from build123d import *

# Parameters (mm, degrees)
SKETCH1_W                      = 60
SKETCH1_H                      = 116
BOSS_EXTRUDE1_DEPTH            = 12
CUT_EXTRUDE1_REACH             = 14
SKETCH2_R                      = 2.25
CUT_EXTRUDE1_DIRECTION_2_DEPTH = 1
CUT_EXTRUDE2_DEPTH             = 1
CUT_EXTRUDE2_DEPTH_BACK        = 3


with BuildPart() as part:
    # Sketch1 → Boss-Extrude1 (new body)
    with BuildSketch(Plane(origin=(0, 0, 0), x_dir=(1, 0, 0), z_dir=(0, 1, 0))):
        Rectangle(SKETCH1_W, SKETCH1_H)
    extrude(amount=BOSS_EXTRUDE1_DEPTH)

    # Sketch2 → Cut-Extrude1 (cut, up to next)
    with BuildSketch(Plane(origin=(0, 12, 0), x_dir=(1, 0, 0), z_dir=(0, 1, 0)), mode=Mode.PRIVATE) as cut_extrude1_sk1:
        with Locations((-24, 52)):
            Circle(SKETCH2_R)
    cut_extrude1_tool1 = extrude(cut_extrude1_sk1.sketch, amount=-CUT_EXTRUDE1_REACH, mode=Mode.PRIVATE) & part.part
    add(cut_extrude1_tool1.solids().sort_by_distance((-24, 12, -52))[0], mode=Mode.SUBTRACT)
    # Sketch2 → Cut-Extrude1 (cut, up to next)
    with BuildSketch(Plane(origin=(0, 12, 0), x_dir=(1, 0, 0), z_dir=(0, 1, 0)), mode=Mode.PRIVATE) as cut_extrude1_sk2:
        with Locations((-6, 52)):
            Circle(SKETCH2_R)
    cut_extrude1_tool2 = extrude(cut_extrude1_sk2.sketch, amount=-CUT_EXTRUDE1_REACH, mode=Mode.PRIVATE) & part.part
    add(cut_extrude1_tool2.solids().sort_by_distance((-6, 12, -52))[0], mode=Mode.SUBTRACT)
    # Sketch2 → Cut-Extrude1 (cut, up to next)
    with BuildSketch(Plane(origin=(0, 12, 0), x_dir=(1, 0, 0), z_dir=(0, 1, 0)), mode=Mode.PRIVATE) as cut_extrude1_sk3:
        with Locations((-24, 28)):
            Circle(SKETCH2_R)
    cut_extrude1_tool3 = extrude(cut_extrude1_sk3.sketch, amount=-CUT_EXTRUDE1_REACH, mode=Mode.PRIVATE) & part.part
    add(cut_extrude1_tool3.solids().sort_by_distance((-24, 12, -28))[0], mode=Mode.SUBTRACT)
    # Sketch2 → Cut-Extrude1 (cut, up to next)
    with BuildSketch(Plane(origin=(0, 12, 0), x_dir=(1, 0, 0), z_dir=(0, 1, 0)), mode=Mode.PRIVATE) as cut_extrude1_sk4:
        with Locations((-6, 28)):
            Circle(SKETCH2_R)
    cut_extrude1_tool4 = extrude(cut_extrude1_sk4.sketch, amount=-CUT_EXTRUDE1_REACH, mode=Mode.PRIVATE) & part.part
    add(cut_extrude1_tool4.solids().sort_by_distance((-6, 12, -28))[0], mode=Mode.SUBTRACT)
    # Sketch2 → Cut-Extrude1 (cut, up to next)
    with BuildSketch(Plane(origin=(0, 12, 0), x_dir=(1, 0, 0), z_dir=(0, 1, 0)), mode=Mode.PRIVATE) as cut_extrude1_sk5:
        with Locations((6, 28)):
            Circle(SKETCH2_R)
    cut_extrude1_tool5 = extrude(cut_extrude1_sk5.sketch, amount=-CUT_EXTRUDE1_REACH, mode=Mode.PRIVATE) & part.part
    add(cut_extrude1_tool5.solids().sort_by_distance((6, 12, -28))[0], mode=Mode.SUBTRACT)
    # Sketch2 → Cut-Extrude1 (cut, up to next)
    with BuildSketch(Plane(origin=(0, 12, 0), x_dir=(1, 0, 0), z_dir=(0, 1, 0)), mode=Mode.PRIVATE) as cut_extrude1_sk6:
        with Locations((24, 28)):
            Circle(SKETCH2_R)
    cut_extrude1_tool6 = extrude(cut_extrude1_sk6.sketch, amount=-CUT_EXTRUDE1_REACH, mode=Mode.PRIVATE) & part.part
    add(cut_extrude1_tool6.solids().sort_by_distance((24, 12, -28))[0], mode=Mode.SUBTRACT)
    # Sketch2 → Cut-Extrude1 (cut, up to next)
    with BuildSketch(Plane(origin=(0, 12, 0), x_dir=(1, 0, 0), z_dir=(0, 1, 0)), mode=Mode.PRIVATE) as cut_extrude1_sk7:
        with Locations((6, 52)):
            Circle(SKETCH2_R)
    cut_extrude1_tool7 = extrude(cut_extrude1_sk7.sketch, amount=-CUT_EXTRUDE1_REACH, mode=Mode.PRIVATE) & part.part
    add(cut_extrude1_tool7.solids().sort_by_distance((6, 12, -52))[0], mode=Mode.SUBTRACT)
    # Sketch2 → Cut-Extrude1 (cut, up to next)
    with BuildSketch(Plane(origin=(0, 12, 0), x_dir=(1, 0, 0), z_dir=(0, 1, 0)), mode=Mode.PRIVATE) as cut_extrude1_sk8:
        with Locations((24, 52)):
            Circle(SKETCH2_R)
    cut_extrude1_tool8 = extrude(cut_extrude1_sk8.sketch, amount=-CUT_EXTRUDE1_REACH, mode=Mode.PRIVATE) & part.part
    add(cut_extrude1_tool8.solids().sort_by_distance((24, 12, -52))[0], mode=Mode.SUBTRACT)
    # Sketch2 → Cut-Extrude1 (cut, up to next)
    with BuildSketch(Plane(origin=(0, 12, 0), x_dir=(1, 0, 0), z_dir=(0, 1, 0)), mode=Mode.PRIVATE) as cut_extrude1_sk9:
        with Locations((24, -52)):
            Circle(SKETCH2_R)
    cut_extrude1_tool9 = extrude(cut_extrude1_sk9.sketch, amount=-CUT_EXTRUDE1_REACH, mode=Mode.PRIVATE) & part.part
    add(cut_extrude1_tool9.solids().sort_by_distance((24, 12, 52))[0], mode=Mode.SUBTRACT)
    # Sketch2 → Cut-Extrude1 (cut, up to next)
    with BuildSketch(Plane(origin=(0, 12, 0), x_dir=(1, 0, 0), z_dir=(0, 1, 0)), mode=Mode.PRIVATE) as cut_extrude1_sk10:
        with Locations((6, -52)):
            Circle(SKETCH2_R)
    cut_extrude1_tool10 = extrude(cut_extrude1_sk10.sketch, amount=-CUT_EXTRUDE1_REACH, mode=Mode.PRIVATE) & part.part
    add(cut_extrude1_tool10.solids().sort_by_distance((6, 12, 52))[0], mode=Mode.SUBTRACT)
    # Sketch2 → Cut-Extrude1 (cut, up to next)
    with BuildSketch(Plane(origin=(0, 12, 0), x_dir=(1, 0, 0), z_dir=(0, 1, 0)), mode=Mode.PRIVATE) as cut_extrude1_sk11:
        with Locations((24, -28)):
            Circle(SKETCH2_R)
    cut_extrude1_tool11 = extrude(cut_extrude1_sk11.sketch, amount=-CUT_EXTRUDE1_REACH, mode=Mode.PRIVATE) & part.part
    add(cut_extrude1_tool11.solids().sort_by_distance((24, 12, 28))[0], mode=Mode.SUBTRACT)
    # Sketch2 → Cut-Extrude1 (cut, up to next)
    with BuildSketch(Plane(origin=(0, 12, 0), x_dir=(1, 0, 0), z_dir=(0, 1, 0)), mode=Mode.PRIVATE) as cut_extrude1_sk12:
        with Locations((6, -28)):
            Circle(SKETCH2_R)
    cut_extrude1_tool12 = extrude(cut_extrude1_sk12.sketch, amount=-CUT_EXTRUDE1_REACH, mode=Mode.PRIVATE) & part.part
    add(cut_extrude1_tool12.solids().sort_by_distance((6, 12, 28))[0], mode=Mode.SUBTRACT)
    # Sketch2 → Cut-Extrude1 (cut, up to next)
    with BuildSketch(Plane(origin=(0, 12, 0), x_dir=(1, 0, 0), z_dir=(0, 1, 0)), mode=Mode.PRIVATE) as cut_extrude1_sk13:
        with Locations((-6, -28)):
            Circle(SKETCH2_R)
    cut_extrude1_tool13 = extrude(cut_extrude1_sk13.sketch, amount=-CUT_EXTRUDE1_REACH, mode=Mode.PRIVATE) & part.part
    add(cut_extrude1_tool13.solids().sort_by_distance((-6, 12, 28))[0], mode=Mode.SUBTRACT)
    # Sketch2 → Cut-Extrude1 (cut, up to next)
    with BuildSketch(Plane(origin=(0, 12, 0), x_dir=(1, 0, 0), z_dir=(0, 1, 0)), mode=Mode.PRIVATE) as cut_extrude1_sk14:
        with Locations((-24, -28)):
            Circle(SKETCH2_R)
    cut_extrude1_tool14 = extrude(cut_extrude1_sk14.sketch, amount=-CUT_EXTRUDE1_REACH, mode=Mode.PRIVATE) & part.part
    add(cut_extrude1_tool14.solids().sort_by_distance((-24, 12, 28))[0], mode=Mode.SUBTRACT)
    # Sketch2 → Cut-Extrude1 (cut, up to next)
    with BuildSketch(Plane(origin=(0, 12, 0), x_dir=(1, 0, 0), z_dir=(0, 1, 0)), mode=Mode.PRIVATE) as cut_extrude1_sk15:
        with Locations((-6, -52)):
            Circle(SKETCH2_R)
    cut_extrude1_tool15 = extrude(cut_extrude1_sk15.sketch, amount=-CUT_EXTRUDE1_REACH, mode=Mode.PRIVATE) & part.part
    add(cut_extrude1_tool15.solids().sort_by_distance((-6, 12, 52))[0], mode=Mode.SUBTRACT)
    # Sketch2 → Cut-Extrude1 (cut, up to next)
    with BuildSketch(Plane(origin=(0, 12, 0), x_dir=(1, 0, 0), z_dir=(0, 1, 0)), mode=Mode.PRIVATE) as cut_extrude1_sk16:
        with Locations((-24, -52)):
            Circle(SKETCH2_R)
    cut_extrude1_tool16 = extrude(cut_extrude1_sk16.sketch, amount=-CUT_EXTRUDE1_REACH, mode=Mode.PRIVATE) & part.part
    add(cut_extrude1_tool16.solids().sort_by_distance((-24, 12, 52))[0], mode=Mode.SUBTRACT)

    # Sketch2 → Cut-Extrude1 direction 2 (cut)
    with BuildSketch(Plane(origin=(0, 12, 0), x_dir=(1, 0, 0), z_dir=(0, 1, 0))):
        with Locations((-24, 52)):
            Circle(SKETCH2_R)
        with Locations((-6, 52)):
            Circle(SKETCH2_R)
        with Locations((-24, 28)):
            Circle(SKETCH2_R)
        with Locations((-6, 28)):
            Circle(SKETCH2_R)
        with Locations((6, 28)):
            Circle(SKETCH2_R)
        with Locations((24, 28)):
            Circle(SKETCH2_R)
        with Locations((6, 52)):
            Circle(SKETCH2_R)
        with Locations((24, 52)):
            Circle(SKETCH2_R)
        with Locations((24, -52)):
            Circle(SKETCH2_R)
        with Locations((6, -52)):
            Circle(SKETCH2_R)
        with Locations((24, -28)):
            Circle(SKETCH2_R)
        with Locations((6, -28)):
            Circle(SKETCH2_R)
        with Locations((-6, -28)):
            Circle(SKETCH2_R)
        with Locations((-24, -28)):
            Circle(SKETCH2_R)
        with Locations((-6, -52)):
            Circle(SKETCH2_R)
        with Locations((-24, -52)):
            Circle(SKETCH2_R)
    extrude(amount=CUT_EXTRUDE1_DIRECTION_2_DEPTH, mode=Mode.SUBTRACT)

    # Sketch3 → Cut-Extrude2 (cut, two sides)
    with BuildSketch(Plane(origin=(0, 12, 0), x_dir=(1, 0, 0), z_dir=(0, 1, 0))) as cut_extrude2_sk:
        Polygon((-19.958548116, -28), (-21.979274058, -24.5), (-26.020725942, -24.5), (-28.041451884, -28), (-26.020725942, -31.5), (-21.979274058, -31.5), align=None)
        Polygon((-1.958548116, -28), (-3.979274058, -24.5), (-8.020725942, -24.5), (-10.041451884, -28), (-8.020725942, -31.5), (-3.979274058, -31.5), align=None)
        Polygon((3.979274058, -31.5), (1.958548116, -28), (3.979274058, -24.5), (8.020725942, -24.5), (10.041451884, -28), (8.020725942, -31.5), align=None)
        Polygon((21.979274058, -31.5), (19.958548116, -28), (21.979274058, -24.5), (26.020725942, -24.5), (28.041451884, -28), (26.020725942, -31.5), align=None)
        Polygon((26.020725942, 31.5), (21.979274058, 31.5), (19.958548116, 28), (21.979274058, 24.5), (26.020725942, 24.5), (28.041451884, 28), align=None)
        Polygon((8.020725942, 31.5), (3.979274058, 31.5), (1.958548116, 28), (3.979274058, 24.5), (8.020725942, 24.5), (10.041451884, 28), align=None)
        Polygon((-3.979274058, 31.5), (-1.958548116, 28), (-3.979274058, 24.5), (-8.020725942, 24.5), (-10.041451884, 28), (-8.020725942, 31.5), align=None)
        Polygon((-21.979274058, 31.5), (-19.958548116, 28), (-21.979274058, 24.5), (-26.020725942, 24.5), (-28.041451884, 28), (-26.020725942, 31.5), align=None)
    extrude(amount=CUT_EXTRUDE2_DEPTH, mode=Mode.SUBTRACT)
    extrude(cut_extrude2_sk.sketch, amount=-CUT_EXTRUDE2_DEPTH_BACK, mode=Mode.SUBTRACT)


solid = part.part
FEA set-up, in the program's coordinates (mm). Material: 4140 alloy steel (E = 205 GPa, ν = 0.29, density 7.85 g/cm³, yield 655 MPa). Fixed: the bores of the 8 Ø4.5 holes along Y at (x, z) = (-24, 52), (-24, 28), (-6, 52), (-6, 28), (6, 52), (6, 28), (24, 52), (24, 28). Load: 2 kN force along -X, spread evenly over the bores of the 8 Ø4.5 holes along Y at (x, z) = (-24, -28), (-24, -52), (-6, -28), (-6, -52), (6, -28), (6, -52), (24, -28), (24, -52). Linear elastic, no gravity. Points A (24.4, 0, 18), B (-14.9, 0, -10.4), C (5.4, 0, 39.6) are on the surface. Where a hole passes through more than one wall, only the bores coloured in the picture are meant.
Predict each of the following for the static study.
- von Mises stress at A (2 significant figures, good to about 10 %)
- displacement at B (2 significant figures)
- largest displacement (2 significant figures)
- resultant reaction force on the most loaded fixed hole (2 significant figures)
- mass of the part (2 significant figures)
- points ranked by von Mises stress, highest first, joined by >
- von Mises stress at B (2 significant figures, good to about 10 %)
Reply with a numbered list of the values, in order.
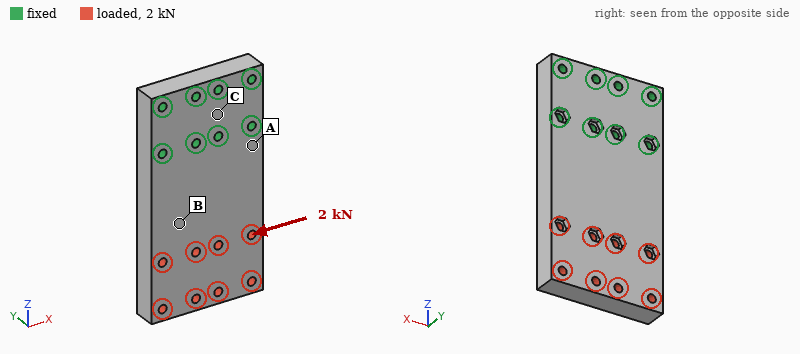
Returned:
1. 17 MPa
2. 4.1 µm
3. 12 µm
4. 2.4 kN
5. 630 g
6. A > B > C
7. 7.7 MPa
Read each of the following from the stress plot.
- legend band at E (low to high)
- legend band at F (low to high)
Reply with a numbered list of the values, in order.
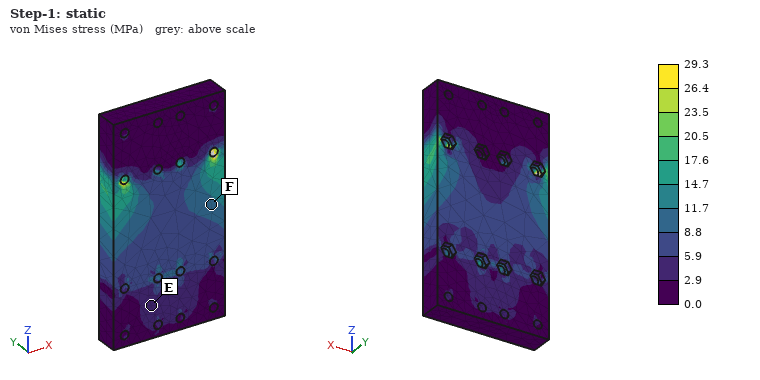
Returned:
1. 2.9 to 5.9 MPa
2. 8.8 to 11.7 MPa
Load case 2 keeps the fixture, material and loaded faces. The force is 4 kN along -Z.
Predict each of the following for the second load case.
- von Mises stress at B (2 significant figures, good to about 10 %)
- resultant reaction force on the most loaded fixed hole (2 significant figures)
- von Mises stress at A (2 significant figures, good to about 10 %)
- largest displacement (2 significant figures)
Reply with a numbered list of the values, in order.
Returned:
1. 7.3 MPa
2. 950 N
3. 7.6 MPa
4. 3.9 µm
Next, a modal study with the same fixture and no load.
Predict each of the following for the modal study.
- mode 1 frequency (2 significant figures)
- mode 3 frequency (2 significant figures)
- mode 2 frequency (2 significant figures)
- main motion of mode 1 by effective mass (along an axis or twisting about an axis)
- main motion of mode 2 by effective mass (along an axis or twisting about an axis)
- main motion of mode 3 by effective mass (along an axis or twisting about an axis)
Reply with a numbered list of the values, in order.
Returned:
1. 1300 Hz
2. 5100 Hz
3. 3900 Hz
4. along Y
5. twisting about Z
6. along X
